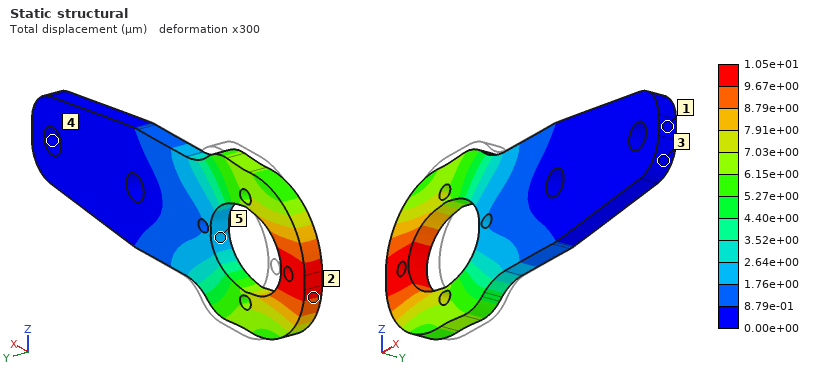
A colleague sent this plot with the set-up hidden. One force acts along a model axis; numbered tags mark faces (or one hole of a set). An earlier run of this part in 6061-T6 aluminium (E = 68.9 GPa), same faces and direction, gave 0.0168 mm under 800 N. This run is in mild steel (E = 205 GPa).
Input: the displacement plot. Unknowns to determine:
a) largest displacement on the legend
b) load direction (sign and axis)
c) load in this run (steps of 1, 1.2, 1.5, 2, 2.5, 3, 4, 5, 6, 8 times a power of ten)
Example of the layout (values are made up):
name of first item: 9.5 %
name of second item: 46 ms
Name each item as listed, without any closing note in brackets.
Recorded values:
largest displacement on the legend: 1.05e+01 µm
load direction: -X
load in this run: 1.5 kN
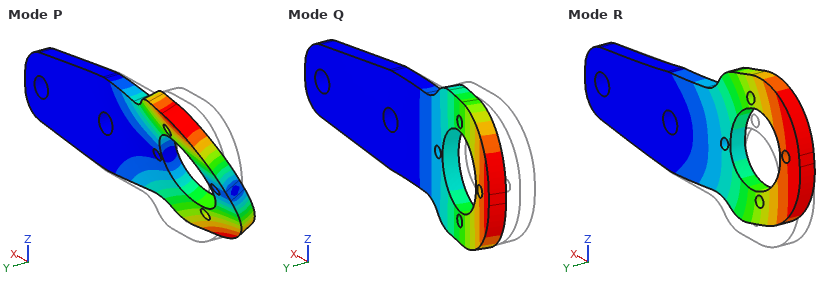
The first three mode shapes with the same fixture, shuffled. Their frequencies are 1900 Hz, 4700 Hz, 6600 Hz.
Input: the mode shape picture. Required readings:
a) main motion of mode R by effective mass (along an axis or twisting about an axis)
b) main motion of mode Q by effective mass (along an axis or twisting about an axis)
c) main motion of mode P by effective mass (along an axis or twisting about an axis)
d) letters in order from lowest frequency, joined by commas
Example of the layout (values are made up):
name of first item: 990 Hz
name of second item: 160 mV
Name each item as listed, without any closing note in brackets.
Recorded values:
main motion of mode R by effective mass: along Z
main motion of mode Q by effective mass: along Y
main motion of mode P by effective mass: twisting about X
letters in order from lowest frequency, joined by commas: Q, P, R
